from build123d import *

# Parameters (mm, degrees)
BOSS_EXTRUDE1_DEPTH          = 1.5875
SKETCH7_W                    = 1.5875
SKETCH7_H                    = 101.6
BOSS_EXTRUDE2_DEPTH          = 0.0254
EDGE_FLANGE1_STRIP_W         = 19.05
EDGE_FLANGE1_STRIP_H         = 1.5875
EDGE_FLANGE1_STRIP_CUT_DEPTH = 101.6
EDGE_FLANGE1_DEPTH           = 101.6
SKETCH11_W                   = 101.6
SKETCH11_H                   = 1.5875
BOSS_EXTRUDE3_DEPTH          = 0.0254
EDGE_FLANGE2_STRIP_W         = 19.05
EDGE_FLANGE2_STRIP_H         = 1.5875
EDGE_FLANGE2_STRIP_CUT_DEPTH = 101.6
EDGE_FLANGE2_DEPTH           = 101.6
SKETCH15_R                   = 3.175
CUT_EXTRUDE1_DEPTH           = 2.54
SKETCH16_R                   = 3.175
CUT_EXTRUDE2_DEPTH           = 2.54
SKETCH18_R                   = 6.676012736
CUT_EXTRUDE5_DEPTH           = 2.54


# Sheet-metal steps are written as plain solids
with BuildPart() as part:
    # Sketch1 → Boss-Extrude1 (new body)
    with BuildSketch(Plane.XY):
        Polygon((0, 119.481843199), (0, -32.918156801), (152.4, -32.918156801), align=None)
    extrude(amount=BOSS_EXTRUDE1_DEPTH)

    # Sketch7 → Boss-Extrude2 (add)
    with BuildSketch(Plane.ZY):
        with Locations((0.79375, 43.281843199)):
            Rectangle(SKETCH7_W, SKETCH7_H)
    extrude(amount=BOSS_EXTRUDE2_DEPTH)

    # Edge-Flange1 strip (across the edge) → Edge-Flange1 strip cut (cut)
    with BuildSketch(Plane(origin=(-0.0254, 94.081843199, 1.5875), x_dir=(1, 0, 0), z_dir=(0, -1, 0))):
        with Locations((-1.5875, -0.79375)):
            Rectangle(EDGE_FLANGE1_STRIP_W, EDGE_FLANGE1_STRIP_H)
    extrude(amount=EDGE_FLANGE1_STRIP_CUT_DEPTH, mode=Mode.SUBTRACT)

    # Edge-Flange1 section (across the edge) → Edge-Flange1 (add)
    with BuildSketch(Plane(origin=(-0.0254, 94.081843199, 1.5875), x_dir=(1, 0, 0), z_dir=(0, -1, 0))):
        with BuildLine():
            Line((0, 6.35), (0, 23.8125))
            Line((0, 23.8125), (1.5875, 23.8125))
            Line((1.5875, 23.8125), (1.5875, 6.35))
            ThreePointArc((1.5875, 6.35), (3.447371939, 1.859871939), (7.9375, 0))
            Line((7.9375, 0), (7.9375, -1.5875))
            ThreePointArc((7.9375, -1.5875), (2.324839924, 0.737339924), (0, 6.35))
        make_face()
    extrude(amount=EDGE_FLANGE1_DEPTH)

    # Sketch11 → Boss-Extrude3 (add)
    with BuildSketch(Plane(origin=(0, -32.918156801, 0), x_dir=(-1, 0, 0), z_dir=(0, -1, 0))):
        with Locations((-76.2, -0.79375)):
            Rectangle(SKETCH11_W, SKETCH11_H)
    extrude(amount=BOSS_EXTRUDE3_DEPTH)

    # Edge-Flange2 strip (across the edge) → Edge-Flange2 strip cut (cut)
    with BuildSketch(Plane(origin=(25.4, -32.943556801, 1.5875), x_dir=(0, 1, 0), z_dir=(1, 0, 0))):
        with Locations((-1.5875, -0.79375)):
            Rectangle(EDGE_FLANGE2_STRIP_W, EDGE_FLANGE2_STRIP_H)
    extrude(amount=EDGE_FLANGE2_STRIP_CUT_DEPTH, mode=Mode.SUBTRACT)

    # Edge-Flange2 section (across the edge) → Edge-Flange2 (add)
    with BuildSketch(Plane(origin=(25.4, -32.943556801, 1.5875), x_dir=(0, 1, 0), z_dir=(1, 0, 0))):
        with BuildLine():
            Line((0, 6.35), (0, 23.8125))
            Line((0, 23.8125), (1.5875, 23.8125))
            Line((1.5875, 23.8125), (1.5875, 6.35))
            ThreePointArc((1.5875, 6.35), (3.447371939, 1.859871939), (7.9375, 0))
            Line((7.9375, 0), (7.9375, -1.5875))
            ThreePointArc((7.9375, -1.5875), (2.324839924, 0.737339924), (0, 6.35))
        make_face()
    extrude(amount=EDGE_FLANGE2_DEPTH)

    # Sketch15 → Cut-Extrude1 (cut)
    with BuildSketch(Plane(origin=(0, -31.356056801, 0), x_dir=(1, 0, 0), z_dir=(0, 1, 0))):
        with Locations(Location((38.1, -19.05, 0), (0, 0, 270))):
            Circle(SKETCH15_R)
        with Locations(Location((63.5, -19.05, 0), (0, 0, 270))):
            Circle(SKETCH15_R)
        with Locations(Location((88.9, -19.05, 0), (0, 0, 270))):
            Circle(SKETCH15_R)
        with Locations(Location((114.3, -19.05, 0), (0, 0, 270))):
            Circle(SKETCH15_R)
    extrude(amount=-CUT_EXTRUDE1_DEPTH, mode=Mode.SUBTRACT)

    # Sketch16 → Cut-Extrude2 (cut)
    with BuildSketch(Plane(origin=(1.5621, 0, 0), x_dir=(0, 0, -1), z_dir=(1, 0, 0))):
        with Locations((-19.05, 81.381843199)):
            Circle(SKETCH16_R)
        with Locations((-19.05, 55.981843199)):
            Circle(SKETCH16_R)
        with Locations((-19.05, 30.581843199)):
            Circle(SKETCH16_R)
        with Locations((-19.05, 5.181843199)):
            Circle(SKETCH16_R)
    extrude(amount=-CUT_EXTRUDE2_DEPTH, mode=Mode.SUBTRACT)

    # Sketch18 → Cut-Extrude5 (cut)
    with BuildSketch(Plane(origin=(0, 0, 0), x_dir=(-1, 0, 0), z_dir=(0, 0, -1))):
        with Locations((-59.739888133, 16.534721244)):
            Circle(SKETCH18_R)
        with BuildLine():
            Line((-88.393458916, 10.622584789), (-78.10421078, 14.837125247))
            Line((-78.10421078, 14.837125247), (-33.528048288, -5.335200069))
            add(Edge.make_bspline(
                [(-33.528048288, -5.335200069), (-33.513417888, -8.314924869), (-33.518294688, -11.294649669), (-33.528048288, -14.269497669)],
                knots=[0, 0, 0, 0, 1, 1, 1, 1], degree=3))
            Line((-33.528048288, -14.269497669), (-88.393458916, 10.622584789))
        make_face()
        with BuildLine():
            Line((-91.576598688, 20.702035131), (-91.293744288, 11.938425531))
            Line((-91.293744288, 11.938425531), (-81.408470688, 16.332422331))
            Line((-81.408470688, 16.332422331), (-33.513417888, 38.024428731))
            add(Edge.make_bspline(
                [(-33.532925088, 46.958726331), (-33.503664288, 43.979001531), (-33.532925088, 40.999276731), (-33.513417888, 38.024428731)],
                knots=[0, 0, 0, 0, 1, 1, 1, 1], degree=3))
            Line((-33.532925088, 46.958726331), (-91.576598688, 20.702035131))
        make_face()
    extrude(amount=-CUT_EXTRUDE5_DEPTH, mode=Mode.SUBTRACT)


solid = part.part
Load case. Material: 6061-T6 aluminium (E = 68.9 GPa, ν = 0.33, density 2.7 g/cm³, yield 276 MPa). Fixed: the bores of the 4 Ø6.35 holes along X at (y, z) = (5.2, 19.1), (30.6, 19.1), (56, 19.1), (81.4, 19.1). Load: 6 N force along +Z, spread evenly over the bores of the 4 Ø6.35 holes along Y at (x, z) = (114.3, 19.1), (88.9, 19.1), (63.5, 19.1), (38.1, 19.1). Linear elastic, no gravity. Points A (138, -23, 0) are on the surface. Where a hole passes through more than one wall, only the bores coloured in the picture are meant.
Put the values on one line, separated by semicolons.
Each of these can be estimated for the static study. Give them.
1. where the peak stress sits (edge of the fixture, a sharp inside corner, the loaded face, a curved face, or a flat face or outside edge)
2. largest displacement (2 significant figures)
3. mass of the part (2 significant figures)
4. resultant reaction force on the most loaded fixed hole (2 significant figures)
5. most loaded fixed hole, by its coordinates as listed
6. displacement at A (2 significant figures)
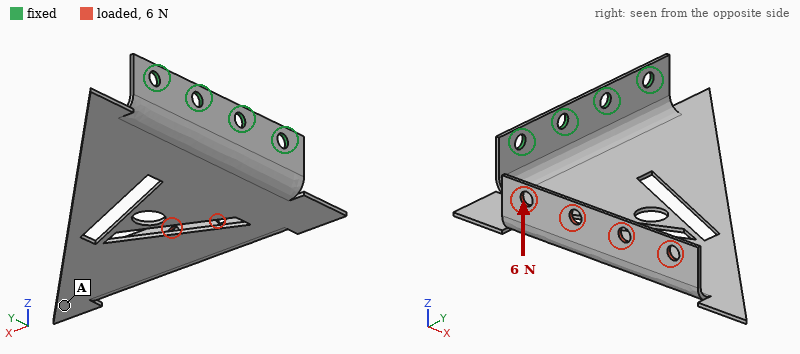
a curved face; 2.3 mm; 62 g; 8.9 N; (5.2, 19.1); 2.0 mm
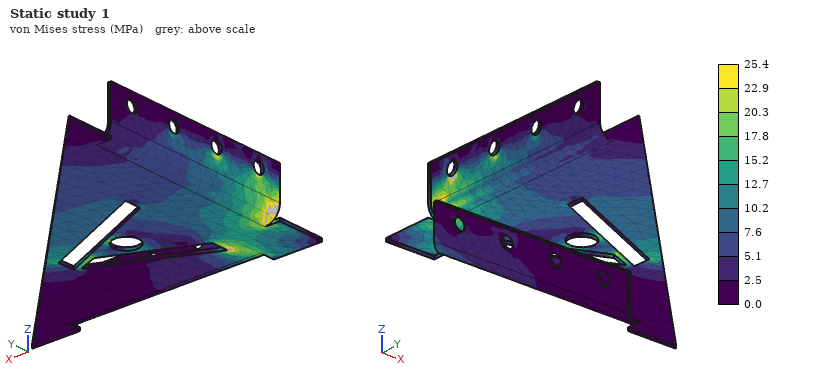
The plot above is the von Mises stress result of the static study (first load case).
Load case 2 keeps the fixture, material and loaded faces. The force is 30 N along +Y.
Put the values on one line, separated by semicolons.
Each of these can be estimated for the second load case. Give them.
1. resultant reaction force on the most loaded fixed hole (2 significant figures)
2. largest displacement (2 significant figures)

31 N; 2.1 mm
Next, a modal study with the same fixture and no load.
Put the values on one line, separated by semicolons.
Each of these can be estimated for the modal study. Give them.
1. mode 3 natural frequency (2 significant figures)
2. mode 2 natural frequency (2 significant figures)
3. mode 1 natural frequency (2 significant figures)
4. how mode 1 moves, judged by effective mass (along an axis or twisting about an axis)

380 Hz; 270 Hz; 67 Hz; along Z
